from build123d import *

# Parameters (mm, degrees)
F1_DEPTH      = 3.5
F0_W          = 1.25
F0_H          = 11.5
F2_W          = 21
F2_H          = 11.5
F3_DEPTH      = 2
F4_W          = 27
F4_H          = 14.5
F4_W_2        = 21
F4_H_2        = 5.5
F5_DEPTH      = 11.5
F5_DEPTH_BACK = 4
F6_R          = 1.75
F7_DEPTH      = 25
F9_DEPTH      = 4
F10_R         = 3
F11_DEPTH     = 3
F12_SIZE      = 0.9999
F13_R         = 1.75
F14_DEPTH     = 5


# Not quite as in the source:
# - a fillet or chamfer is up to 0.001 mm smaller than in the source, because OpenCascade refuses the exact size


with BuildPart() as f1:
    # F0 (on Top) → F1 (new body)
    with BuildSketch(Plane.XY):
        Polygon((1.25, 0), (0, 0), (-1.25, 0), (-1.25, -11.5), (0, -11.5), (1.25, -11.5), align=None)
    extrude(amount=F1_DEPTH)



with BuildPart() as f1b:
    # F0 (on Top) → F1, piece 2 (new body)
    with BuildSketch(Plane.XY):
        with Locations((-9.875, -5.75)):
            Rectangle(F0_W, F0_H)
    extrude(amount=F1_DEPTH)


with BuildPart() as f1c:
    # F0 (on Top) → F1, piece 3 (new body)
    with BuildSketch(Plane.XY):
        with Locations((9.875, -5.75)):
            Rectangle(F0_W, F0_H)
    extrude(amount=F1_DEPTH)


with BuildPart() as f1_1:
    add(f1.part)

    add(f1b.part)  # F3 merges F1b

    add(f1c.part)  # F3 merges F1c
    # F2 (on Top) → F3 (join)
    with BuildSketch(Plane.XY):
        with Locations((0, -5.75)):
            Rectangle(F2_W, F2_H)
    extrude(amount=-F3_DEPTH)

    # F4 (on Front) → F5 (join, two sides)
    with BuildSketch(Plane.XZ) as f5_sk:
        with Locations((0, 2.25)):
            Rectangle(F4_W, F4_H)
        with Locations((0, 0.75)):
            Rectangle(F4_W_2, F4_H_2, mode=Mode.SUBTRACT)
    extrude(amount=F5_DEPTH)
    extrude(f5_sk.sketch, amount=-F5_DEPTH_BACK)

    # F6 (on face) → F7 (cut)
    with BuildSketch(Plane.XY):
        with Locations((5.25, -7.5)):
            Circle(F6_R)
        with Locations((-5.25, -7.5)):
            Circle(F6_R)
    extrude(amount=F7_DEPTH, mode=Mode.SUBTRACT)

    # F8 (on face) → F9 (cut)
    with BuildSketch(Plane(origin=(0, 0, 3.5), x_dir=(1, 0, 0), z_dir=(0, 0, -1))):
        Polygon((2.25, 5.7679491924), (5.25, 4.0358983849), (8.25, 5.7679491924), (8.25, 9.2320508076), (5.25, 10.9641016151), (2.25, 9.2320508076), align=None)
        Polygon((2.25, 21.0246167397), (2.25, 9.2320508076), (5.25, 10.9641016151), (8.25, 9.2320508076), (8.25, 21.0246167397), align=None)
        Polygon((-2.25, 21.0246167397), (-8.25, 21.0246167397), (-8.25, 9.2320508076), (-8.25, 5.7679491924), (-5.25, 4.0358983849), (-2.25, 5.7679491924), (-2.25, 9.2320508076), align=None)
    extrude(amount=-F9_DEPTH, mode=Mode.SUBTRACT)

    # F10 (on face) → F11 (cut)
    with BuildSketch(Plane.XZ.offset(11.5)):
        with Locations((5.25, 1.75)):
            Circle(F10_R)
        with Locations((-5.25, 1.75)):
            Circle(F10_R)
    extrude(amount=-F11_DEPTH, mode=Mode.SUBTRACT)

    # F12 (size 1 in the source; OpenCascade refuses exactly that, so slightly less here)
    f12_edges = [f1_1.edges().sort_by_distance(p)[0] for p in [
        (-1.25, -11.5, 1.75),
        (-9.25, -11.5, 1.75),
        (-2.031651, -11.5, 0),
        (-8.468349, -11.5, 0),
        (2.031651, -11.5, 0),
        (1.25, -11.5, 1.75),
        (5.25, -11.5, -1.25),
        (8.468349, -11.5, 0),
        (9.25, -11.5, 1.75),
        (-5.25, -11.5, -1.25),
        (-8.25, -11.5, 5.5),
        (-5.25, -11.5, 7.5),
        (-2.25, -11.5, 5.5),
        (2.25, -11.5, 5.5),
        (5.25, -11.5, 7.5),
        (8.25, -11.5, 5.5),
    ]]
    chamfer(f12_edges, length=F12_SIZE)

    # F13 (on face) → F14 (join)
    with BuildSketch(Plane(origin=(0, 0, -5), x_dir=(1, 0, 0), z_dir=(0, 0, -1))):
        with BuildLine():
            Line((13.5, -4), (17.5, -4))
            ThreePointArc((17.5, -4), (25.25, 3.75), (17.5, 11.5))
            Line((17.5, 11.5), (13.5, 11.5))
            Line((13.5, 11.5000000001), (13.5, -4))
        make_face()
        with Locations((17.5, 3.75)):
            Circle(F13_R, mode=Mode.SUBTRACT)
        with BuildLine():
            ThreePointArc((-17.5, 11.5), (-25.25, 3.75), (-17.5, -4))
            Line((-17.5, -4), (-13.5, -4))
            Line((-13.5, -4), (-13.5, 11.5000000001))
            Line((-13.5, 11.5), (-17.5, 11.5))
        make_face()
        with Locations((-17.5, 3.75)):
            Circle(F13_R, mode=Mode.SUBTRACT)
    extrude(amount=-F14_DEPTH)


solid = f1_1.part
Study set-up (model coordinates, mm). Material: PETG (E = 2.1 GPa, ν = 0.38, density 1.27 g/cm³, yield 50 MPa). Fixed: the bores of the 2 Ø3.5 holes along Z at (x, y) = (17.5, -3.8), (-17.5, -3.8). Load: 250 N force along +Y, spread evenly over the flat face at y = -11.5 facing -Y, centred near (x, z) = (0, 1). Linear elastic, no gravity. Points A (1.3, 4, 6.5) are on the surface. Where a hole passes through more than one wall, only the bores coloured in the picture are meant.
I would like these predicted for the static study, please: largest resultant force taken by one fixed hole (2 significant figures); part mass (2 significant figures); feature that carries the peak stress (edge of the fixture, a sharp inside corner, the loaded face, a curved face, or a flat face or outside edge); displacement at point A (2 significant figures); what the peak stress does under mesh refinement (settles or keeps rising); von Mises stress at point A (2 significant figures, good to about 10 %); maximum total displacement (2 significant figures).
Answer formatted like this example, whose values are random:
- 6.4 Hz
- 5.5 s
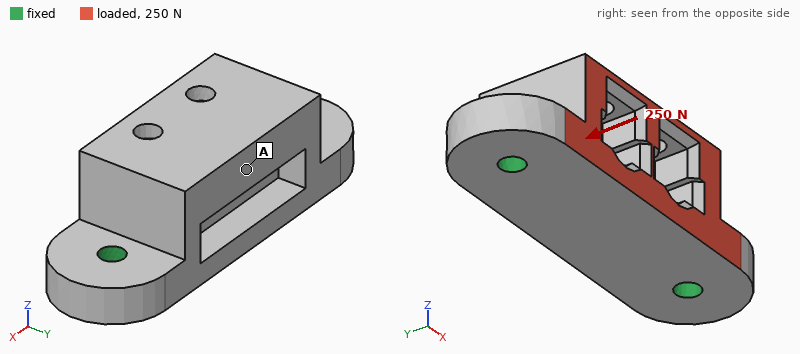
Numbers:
- 130 N
- 7.6 g
- edge of the fixture
- 0.088 mm
- keeps rising
- 1.4 MPa
- 0.11 mm
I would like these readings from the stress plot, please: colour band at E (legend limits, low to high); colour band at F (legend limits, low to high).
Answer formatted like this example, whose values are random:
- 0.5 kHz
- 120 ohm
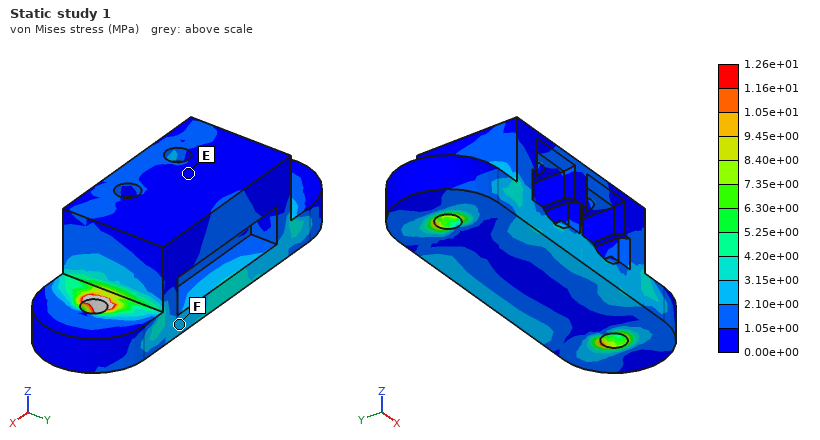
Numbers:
- 0.00e+00 to 1.05e+00 MPa
- 2.10e+00 to 3.15e+00 MPa
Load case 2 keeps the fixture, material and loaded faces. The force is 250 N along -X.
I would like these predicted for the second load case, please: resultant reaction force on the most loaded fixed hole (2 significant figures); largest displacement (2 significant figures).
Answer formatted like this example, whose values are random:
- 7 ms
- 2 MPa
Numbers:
- 140 N
- 58 µm
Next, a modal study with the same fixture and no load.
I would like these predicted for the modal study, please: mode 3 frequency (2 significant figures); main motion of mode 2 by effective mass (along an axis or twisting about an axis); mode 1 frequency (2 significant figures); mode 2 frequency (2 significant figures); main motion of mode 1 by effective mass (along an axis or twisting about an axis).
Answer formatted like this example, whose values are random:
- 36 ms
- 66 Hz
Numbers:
- 6400 Hz
- along Z
- 3100 Hz
- 5100 Hz
- along Y
